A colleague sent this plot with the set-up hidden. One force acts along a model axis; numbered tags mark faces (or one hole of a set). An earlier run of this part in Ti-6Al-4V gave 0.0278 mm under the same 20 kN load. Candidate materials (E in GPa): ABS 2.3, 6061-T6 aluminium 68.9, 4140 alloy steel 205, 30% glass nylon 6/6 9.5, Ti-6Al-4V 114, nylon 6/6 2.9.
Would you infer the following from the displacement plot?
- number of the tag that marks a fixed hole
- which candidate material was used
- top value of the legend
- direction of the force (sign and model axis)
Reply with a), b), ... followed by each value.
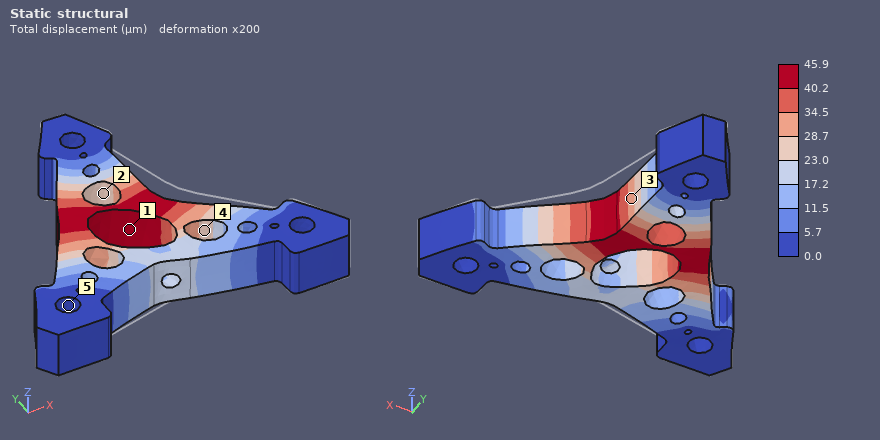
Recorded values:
a) 5
b) 6061-T6 aluminium
c) 45.9 µm
d) -X
